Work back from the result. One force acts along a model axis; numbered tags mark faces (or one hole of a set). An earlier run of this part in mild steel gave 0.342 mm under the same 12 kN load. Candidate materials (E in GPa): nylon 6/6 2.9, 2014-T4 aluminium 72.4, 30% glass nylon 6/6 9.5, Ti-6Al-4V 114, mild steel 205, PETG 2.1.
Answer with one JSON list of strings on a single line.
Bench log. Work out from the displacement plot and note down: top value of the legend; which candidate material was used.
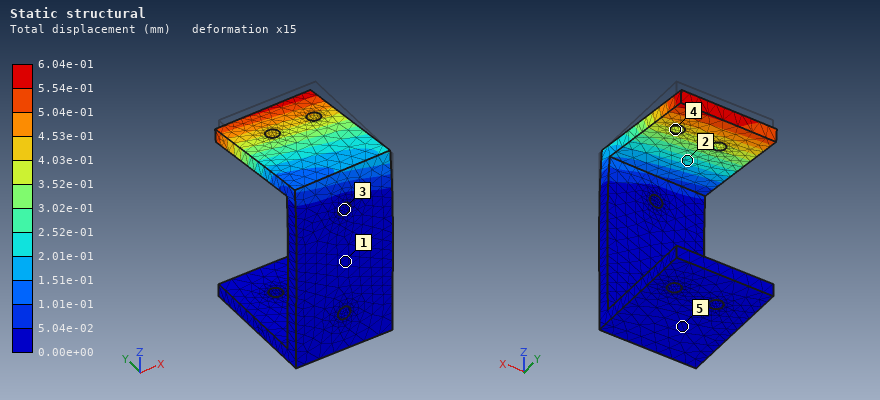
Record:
["6.04e-01 mm", "Ti-6Al-4V"]
